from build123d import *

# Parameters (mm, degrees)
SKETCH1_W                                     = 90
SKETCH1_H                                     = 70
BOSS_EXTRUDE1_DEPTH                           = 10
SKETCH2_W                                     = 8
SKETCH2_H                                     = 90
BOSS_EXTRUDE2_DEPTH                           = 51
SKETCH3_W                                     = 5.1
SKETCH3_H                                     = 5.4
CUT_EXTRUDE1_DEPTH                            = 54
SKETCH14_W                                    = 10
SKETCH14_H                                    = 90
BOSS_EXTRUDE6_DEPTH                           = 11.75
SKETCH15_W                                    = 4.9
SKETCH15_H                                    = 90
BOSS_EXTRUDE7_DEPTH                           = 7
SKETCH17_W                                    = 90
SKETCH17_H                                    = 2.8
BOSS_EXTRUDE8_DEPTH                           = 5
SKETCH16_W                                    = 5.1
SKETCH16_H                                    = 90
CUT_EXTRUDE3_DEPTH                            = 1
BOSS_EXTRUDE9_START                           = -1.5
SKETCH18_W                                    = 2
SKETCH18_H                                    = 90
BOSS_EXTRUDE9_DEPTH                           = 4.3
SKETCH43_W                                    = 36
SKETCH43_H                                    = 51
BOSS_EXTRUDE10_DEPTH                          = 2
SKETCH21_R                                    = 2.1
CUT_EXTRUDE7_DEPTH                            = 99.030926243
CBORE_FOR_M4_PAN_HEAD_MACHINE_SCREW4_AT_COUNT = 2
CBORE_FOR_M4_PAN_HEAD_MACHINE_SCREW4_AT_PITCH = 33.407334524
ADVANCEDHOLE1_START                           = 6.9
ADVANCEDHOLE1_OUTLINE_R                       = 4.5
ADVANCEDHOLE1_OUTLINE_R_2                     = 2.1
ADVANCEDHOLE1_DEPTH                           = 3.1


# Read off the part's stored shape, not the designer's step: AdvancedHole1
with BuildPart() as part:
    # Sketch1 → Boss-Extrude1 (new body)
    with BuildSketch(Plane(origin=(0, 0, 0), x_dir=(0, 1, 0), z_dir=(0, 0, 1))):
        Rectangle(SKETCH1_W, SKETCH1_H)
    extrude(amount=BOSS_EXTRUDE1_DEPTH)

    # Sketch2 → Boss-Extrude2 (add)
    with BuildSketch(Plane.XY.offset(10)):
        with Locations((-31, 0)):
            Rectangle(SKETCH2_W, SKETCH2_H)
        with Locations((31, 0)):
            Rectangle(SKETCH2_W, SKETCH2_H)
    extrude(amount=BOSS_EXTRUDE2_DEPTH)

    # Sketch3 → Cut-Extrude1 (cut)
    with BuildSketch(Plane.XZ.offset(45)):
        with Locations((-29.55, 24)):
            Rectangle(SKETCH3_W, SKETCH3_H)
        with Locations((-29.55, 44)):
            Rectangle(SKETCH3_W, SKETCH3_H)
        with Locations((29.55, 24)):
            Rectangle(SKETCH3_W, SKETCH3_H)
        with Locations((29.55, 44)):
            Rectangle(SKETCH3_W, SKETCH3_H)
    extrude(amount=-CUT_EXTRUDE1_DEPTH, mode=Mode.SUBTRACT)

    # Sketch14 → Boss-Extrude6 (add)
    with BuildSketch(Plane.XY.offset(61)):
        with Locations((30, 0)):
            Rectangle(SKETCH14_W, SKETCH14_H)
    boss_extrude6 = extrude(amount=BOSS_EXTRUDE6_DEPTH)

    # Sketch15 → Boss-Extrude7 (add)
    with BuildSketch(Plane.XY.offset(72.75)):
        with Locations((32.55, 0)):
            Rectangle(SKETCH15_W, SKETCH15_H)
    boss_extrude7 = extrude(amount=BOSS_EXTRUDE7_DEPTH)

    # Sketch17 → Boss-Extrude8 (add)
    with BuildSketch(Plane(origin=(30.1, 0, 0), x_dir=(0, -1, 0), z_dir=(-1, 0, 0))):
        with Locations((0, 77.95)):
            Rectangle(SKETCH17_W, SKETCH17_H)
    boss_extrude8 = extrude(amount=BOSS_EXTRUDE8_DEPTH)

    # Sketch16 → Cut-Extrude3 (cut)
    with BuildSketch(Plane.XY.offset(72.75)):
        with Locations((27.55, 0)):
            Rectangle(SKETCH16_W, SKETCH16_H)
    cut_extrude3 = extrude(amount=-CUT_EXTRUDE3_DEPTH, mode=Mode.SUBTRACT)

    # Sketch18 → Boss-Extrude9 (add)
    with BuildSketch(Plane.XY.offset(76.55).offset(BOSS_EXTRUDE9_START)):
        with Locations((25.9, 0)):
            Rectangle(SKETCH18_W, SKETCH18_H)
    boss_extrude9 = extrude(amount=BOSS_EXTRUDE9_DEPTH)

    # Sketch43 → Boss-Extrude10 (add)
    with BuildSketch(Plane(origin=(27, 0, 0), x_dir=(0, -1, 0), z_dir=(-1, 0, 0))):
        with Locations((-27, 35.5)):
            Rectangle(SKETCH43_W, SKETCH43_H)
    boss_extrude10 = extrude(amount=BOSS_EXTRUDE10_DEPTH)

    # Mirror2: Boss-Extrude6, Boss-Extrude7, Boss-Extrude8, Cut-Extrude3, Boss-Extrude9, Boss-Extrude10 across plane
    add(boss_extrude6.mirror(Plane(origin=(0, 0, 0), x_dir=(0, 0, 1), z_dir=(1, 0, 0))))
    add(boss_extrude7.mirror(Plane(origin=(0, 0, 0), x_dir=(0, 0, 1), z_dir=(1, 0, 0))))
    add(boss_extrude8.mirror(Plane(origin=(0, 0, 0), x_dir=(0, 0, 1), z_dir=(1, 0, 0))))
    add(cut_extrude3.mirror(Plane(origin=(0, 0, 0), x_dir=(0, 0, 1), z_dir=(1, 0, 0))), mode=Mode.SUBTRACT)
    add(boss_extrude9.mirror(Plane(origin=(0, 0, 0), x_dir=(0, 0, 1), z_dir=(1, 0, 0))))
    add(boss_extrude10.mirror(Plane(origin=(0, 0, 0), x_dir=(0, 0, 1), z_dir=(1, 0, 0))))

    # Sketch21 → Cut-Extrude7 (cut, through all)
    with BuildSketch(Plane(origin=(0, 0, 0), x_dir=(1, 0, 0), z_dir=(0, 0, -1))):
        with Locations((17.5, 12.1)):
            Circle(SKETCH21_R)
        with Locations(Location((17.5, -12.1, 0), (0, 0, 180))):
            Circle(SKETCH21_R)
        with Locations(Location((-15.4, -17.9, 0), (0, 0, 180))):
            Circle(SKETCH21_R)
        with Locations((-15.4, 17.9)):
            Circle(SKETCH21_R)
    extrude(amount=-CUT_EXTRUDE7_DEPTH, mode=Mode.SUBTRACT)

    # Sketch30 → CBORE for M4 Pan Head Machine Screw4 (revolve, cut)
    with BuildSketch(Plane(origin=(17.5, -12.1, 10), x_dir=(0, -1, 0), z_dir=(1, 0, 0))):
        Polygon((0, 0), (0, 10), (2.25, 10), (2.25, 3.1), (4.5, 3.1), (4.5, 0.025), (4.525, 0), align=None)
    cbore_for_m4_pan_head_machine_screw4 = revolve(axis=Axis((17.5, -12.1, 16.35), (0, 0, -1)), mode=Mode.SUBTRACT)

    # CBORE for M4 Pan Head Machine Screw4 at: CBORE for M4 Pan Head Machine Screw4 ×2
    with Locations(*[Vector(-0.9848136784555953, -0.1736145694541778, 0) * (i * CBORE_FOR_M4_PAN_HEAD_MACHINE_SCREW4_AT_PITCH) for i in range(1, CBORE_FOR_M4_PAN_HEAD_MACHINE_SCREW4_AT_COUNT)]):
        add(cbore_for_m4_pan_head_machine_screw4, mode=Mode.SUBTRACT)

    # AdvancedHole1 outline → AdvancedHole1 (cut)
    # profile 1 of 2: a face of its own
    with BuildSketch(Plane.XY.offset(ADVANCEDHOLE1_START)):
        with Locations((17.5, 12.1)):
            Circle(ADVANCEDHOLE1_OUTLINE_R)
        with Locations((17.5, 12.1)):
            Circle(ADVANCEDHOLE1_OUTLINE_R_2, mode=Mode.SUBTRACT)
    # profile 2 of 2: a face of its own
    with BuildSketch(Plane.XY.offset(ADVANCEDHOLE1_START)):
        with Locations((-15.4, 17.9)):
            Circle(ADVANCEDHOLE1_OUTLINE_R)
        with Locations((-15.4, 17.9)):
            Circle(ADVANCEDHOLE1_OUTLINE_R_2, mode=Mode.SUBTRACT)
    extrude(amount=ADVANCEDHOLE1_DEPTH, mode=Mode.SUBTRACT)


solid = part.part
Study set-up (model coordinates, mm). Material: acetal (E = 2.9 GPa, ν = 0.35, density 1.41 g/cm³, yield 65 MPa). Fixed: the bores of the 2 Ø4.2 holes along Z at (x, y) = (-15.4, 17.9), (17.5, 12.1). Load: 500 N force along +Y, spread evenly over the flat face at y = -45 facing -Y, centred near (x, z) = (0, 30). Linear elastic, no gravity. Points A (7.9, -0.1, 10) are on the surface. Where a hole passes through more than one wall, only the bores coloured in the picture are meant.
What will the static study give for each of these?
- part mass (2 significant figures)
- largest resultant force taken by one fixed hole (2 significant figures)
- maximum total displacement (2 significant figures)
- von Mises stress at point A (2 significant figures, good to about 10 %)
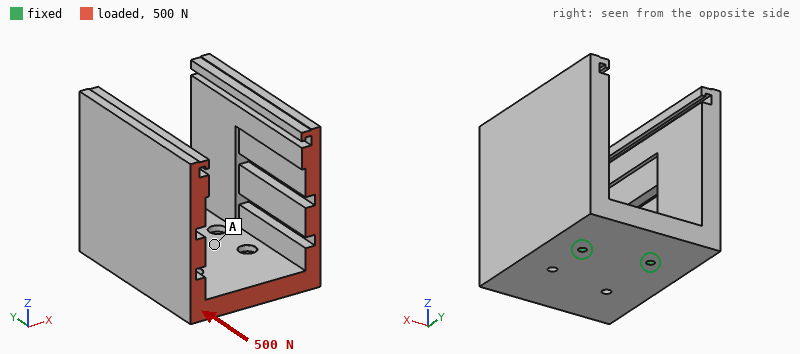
230 g
270 N
1.5 mm
2.8 MPa
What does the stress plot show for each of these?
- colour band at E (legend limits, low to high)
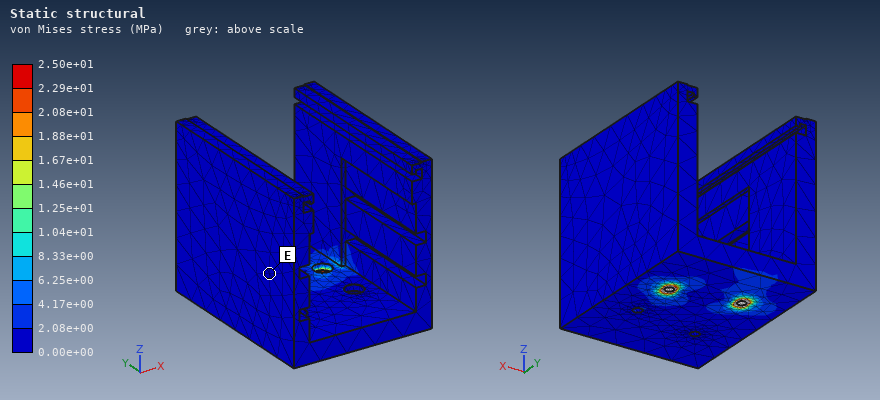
0.00e+00 to 2.08e+00 MPa
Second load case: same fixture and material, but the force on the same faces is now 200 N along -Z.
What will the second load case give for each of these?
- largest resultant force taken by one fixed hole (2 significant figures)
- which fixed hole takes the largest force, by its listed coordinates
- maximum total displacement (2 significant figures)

150 N
(17.5, 12.1)
1.4 mm
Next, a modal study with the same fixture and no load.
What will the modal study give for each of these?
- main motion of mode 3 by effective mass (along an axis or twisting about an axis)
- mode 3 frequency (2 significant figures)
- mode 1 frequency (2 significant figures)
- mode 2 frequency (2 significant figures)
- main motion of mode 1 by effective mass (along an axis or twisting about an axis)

along X
250 Hz
200 Hz
240 Hz
along Y
